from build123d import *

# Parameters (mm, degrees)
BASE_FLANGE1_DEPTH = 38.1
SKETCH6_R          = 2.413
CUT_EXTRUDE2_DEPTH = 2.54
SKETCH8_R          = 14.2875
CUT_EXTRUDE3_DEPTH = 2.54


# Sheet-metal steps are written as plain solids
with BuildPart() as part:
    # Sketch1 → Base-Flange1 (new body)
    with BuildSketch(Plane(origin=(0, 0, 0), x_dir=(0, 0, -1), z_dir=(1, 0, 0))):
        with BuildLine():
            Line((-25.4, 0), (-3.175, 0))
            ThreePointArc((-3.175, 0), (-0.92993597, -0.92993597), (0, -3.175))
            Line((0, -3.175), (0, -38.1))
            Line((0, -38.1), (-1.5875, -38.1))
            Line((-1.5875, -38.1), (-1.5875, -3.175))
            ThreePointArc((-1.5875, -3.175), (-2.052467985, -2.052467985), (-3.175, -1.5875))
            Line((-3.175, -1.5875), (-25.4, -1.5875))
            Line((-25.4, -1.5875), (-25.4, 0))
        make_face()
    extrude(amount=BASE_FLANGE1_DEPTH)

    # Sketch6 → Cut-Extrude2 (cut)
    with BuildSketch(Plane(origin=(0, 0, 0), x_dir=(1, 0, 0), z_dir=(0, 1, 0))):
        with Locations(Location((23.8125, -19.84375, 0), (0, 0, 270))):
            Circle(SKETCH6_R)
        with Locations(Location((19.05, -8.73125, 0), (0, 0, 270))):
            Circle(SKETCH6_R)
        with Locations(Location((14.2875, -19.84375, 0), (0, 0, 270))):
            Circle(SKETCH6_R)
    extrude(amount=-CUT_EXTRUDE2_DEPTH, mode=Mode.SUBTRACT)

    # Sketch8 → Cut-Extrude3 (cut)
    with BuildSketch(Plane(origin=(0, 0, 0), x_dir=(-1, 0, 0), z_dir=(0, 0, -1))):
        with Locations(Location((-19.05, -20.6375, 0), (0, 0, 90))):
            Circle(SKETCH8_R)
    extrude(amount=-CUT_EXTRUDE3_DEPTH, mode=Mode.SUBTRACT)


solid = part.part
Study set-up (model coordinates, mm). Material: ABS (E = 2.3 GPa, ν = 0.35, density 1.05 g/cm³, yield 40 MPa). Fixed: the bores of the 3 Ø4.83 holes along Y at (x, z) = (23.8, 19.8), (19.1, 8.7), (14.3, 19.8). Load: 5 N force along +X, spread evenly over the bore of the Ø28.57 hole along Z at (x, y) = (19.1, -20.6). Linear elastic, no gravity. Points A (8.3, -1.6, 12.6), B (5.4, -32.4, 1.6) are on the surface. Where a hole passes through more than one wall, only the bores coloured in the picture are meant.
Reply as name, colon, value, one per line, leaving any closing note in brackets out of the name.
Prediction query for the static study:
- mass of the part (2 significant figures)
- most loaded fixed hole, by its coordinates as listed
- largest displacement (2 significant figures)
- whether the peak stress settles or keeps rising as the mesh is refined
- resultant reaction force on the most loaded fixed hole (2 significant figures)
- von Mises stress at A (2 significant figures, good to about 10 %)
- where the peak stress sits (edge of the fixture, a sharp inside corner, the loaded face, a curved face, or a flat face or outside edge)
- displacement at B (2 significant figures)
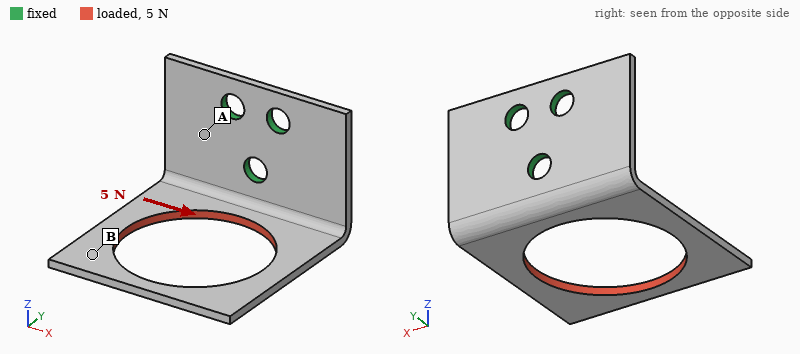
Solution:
mass of the part: 2.7 g
most loaded fixed hole, by its coordinates as listed: (19.1, 8.7)
largest displacement: 0.65 mm
whether the peak stress settles or keeps rising as the mesh is refined: keeps rising
resultant reaction force on the most loaded fixed hole: 5.1 N
von Mises stress at A: 2.1 MPa
where the peak stress sits: edge of the fixture
displacement at B: 0.53 mm
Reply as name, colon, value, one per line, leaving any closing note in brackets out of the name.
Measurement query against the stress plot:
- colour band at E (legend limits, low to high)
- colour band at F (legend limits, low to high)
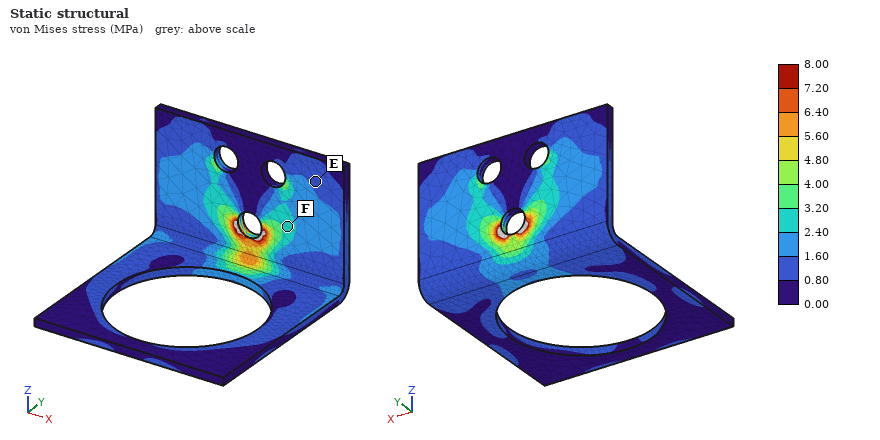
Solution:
colour band at E: 0.80 to 1.60 MPa
colour band at F: 2.40 to 3.20 MPa
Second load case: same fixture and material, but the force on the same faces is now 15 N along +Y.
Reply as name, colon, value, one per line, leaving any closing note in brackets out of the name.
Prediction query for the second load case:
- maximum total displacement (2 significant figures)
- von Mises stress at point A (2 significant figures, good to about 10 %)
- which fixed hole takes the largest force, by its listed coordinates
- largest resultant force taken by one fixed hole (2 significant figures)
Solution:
maximum total displacement: 0.57 mm
von Mises stress at point A: 1.7 MPa
which fixed hole takes the largest force, by its listed coordinates: (19.1, 8.7)
largest resultant force taken by one fixed hole: 18 N
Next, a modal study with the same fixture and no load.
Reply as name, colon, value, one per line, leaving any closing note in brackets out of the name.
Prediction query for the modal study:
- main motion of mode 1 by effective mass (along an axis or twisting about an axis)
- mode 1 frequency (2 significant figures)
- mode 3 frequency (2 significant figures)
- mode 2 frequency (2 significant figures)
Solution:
main motion of mode 1 by effective mass: along Z
mode 1 frequency: 210 Hz
mode 3 frequency: 520 Hz
mode 2 frequency: 400 Hz
